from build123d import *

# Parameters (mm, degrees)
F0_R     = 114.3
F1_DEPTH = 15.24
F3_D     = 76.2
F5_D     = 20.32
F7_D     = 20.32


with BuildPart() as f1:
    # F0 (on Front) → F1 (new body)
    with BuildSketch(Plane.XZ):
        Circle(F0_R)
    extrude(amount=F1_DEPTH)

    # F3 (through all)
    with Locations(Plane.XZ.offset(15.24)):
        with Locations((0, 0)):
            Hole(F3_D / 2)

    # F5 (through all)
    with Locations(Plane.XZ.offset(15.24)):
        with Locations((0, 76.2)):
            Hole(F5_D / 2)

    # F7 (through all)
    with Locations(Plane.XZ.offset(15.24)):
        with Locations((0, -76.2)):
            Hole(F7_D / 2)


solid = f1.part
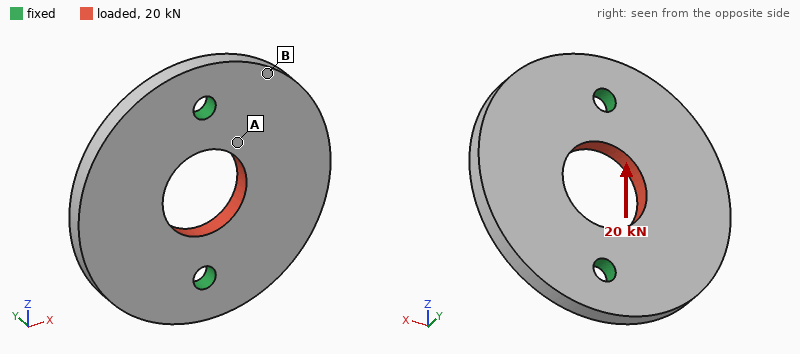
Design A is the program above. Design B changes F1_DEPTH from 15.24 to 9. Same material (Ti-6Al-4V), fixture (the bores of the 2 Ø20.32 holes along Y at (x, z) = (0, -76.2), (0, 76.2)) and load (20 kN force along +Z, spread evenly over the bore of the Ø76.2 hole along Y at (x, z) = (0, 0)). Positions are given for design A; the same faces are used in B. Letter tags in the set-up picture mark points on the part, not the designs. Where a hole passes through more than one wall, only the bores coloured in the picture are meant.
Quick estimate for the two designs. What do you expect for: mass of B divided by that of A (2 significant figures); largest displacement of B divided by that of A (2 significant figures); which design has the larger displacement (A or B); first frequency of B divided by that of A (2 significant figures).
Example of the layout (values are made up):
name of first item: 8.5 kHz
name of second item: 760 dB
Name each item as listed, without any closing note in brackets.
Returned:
mass of B divided by that of A: 0.59
largest displacement of B divided by that of A: 1.7
which design has the larger displacement: B
first frequency of B divided by that of A: 0.62
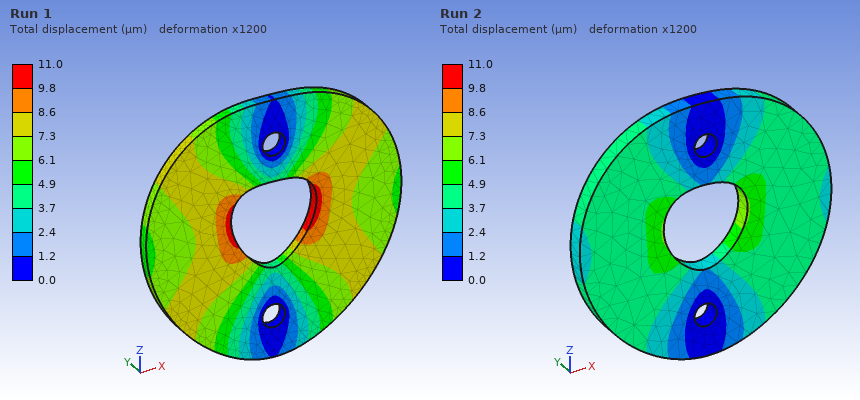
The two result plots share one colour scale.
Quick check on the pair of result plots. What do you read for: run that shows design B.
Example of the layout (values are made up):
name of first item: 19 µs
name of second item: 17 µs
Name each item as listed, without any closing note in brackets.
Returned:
run that shows design B: Run 1
